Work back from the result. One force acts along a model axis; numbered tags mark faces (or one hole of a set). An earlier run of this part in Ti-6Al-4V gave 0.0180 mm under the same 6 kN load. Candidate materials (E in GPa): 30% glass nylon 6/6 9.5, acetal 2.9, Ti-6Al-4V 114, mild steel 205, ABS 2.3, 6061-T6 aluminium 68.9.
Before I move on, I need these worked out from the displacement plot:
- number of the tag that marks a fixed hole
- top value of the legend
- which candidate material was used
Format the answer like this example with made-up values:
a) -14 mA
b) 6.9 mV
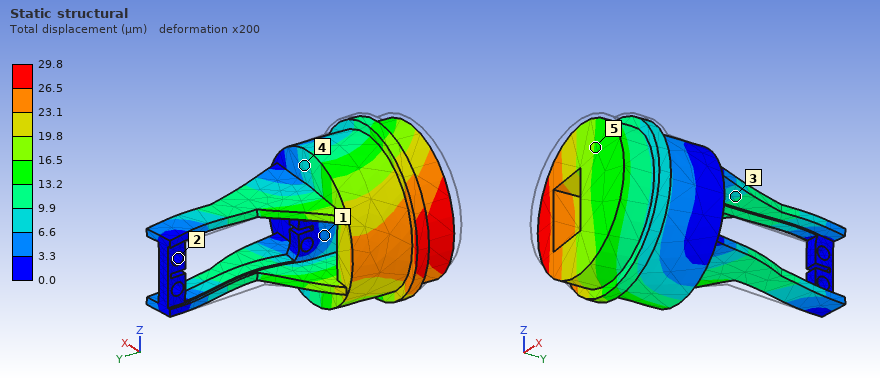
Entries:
a) 2
b) 29.8 µm
c) 6061-T6 aluminium
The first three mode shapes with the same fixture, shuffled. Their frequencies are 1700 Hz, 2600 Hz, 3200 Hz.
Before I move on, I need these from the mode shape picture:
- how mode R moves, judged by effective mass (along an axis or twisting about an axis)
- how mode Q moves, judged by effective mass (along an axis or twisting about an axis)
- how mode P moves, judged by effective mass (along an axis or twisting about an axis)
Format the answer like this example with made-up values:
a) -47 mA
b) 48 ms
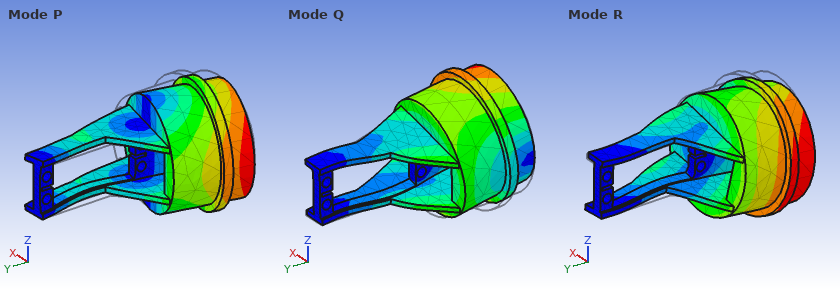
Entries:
a) along Z
b) along Z
c) along X
